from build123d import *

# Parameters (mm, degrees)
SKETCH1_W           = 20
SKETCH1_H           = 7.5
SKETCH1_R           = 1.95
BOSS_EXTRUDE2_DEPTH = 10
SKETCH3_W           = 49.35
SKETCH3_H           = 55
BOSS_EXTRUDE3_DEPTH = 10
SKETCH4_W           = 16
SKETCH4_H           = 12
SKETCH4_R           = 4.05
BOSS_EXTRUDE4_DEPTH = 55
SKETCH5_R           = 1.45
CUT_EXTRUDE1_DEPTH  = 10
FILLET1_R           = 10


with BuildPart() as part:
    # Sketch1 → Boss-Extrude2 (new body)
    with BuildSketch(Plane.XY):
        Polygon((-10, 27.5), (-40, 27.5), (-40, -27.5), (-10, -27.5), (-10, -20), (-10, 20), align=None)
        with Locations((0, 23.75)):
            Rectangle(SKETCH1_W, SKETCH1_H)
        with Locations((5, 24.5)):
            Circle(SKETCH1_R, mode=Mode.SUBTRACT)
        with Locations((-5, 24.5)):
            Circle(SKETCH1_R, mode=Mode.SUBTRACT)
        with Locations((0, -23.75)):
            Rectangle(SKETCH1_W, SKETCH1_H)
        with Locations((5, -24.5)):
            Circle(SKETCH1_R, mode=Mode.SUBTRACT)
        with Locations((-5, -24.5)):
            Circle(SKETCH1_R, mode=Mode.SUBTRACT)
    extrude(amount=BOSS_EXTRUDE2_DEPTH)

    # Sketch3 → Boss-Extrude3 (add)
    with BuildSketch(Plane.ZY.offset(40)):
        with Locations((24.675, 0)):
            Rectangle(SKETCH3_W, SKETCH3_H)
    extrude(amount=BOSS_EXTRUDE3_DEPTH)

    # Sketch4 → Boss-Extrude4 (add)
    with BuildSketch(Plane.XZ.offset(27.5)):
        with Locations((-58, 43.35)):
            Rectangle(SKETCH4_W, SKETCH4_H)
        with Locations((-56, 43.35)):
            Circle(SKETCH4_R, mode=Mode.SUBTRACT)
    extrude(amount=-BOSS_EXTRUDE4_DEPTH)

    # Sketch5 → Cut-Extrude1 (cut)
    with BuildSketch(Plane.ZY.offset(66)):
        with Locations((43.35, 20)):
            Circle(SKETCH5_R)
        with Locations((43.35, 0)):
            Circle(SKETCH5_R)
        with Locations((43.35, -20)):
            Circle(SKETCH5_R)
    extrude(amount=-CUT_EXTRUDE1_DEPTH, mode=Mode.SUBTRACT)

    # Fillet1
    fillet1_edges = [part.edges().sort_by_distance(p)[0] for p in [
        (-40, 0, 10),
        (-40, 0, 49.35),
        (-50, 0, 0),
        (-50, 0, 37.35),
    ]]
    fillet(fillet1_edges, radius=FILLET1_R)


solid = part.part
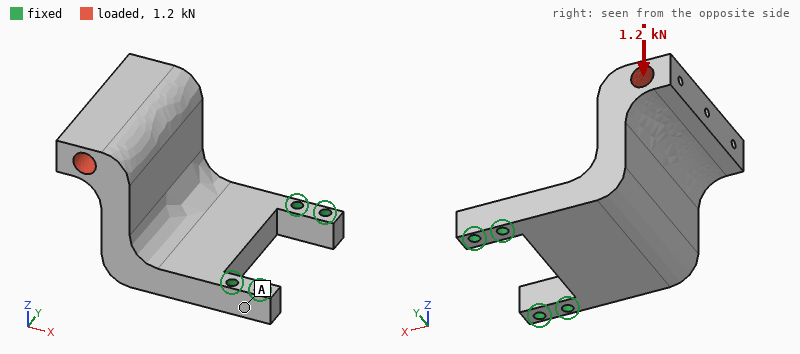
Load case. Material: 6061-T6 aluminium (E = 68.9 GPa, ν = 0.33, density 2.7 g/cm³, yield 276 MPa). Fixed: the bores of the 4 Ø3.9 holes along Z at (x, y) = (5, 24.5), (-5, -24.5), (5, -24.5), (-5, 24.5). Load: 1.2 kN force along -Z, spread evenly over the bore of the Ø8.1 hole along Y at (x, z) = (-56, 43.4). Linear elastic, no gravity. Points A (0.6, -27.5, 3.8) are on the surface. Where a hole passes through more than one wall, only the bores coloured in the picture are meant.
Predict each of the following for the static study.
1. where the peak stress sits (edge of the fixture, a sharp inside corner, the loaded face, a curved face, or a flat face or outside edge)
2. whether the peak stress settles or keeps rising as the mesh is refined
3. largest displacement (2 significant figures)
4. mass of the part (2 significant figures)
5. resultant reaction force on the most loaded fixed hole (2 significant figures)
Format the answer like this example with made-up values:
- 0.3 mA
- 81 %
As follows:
- edge of the fixture
- keeps rising
- 0.65 mm
- 150 g
- 720 N
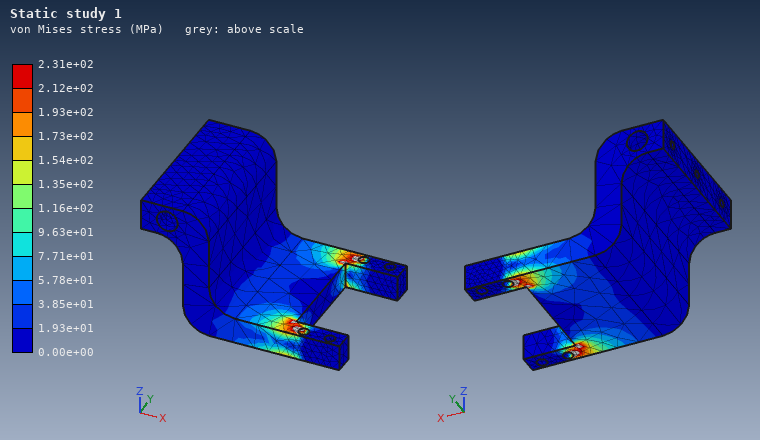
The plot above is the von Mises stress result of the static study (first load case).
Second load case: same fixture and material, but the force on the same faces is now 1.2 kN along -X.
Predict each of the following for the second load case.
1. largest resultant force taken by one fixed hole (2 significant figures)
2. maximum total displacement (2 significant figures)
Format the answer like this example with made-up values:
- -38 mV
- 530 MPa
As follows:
- 620 N
- 0.65 mm
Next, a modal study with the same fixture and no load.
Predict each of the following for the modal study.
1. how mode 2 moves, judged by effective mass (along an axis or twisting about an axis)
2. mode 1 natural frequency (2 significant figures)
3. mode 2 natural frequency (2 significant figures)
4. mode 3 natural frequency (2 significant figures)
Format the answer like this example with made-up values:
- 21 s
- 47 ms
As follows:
- along Y
- 840 Hz
- 2300 Hz
- 3800 Hz
